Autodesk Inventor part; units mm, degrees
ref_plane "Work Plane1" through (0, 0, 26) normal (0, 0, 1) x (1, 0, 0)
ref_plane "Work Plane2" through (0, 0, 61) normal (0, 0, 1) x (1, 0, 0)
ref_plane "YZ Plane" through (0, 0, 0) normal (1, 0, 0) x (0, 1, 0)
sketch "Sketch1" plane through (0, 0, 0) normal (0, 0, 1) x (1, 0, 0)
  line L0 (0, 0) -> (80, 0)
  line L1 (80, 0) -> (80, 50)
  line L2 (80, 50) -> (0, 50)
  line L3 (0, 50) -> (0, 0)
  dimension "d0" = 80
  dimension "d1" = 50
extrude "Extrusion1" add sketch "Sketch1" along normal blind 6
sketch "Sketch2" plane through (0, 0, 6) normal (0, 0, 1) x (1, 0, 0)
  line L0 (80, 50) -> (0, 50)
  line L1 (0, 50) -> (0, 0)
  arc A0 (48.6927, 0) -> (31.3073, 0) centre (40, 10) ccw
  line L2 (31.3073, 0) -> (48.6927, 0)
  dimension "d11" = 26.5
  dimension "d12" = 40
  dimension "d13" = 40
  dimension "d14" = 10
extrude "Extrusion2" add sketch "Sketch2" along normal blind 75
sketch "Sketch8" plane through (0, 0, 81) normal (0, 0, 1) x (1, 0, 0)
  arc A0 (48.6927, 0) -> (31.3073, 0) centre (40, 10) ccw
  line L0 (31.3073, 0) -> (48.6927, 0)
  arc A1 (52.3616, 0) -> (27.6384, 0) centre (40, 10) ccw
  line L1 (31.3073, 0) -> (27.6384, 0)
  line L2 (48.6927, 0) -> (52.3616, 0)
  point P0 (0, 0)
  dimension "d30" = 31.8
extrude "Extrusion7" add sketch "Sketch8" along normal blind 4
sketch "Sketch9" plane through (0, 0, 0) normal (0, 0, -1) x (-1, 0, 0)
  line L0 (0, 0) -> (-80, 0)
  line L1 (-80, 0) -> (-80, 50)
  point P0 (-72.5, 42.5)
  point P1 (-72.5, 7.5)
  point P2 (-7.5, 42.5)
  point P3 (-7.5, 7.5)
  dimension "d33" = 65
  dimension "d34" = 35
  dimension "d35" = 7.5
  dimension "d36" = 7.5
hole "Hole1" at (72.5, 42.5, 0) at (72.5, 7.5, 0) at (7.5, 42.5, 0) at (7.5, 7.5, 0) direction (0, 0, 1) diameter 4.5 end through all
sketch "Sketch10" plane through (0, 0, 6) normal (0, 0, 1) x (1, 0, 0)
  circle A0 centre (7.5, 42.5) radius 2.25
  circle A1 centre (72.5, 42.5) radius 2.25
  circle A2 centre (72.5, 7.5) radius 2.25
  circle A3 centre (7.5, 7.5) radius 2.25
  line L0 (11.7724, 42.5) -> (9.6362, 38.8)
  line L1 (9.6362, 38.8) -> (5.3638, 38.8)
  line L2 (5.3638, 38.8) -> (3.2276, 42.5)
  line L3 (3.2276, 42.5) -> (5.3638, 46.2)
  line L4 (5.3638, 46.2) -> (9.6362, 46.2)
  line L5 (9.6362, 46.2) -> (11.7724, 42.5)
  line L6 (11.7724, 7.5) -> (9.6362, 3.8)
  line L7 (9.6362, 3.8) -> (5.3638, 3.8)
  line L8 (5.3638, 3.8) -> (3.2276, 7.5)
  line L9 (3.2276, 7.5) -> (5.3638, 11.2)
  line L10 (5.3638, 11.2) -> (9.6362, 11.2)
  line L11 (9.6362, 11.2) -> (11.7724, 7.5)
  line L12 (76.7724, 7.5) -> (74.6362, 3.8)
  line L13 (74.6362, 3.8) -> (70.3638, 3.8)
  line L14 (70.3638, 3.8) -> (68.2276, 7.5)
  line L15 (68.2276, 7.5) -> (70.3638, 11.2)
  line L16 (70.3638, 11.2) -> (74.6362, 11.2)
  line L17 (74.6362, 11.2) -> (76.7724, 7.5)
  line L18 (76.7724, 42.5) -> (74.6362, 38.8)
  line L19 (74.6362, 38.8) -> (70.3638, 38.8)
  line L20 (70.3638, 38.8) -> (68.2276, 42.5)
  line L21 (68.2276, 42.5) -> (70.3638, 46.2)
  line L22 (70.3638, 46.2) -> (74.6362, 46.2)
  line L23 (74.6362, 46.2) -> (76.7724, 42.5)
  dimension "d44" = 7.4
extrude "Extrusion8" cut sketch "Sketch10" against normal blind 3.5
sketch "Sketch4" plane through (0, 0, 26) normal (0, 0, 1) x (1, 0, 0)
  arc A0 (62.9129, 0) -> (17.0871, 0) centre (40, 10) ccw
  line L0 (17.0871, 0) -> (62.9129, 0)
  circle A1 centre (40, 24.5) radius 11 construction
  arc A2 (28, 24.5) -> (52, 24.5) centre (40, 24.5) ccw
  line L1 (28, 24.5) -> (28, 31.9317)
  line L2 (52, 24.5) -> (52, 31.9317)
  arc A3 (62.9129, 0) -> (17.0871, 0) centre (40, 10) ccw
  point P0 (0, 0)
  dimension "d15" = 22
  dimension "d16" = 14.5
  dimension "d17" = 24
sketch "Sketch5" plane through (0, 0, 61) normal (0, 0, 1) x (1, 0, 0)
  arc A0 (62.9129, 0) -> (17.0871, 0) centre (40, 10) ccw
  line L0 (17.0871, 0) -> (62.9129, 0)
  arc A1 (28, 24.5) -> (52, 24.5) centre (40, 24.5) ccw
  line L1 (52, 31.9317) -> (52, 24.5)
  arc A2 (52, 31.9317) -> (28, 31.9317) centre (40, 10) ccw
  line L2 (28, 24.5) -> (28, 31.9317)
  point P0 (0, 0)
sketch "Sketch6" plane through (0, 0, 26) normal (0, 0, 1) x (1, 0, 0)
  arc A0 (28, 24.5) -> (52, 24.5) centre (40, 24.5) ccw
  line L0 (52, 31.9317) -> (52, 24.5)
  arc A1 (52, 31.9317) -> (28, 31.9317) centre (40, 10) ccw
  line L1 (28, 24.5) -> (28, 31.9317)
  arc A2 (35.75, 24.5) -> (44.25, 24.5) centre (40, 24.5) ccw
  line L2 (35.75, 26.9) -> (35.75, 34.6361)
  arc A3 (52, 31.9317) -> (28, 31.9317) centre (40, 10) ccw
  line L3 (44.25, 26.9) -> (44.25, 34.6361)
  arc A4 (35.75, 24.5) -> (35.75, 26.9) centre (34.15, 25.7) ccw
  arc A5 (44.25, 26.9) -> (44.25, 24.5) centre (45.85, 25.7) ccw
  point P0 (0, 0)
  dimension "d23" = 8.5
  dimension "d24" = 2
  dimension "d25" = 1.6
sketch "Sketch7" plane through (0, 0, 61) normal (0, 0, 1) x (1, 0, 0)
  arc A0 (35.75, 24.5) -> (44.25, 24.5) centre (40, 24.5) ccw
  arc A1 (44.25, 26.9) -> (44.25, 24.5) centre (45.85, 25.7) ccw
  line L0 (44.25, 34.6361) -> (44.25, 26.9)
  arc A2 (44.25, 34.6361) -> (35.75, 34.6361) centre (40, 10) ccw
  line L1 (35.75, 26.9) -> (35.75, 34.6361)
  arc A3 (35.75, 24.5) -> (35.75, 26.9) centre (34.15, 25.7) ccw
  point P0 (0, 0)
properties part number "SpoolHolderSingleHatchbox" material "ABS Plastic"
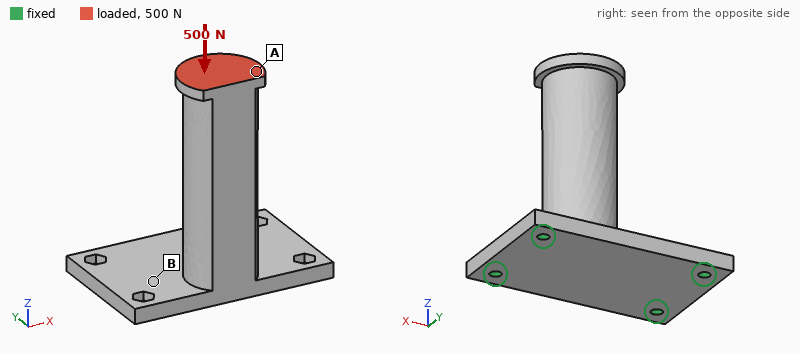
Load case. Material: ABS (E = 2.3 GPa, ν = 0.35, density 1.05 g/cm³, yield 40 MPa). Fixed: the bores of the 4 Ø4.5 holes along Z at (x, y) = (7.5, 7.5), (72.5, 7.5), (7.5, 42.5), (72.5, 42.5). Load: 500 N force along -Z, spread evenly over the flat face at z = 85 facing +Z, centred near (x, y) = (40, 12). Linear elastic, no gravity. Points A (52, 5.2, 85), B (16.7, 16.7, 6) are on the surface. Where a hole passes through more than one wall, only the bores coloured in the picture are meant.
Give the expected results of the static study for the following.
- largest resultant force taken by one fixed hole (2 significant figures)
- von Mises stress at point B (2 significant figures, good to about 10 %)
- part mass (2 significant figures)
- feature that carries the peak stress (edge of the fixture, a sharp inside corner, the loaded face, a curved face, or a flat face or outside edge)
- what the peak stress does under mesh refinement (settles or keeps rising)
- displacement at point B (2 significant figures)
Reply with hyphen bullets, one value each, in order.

- 370 N
- 5.9 MPa
- 68 g
- edge of the fixture
- keeps rising
- 0.18 mm
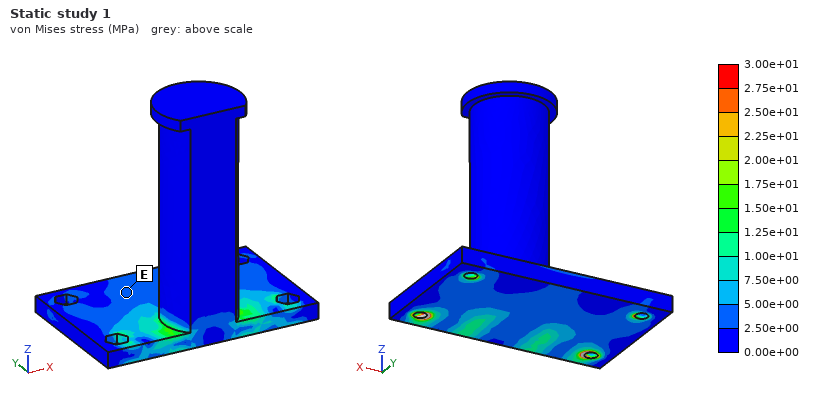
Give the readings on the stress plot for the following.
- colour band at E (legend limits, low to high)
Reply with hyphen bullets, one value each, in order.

- 2.50e+00 to 5.00e+00 MPa
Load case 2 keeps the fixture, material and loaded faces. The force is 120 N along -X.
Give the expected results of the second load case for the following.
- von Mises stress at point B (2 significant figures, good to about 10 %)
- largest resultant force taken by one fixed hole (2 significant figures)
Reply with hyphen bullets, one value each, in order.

- 4.4 MPa
- 170 N
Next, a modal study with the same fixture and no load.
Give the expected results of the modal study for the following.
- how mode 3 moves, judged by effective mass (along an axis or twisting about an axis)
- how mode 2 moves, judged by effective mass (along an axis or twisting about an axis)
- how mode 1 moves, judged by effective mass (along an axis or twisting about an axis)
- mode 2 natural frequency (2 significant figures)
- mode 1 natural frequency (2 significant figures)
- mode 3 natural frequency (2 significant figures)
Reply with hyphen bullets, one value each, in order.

- along Z
- along X
- along Y
- 390 Hz
- 250 Hz
- 800 Hz
